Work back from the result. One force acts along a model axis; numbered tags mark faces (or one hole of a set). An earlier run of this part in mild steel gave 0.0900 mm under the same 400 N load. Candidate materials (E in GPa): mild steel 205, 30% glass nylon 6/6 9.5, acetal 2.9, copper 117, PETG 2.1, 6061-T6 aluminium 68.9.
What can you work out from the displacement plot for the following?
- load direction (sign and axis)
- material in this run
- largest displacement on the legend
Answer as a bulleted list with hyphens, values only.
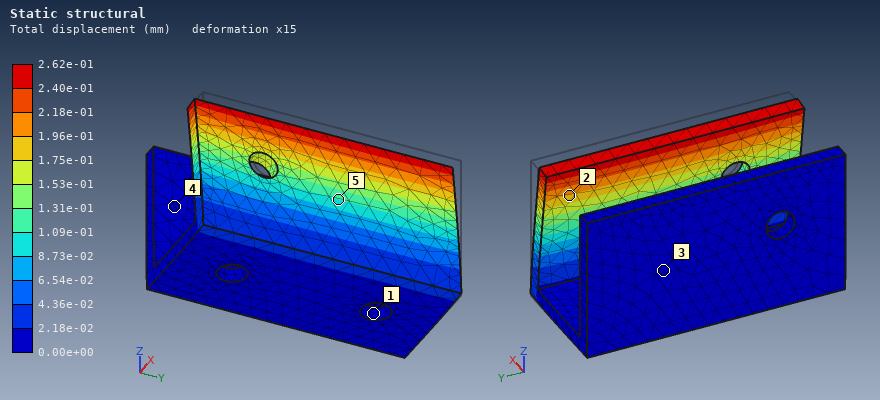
- -X
- 6061-T6 aluminium
- 2.62e-01 mm
